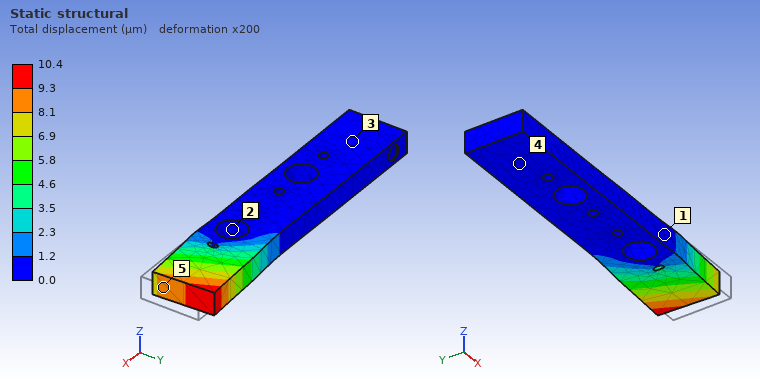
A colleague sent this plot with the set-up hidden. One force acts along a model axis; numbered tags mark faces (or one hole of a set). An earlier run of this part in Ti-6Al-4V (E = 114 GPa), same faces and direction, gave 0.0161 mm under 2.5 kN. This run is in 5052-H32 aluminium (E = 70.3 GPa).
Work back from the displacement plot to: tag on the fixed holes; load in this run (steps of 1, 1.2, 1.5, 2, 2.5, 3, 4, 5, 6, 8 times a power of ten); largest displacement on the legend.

2
1 kN
10.4 µm
